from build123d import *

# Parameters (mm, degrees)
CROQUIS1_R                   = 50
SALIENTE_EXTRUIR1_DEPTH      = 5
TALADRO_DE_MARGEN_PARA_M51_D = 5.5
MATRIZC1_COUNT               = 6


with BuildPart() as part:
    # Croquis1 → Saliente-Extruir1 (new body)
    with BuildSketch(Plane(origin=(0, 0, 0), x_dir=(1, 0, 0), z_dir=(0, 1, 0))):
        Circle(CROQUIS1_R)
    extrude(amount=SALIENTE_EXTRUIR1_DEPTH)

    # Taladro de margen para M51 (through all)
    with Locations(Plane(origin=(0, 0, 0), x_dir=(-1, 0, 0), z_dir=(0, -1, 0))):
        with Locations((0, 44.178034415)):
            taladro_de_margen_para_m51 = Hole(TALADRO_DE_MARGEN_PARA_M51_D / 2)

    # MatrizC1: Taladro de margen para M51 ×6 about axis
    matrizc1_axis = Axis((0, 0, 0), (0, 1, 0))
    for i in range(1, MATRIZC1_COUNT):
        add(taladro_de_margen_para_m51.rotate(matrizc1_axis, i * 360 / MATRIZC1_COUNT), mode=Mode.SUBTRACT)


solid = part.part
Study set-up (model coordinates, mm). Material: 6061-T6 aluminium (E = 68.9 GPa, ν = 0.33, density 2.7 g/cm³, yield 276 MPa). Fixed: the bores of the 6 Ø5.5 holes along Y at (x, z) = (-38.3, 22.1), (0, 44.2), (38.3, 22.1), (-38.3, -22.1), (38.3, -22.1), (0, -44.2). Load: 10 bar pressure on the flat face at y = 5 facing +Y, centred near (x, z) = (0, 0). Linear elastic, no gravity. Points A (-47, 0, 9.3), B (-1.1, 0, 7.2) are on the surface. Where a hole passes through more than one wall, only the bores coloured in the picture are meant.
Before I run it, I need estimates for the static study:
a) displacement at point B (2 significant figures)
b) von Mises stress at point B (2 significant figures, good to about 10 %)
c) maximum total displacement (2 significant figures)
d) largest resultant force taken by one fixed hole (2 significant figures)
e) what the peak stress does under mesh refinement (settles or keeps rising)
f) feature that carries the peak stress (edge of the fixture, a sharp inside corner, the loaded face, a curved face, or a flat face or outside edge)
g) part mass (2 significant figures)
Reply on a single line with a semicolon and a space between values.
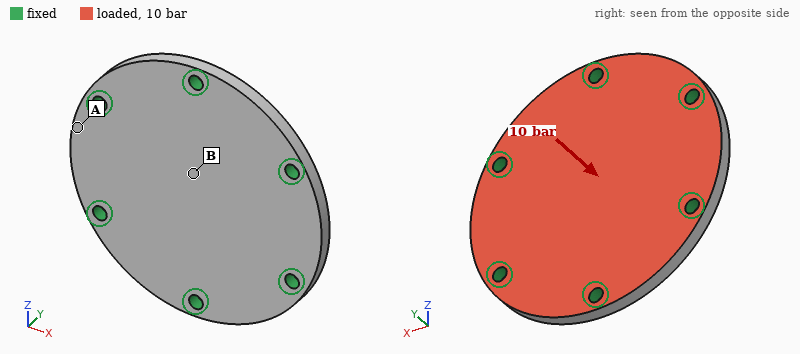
95 µm; 41 MPa; 99 µm; 1.3 kN; keeps rising; edge of the fixture; 100 g
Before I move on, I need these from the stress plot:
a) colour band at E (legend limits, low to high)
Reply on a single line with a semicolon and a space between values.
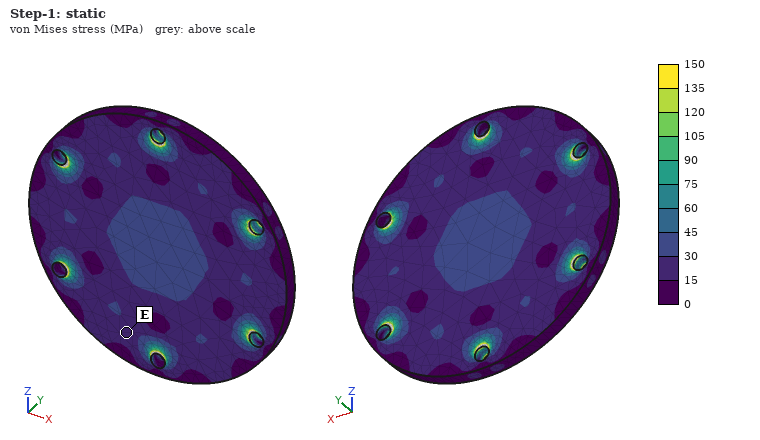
15 to 30 MPa
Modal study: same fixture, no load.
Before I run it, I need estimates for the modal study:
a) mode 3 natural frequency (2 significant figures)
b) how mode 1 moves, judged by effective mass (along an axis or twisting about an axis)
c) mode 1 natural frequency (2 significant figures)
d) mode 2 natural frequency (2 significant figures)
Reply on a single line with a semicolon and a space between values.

11 kHz; along Y; 5400 Hz; 11 kHz
